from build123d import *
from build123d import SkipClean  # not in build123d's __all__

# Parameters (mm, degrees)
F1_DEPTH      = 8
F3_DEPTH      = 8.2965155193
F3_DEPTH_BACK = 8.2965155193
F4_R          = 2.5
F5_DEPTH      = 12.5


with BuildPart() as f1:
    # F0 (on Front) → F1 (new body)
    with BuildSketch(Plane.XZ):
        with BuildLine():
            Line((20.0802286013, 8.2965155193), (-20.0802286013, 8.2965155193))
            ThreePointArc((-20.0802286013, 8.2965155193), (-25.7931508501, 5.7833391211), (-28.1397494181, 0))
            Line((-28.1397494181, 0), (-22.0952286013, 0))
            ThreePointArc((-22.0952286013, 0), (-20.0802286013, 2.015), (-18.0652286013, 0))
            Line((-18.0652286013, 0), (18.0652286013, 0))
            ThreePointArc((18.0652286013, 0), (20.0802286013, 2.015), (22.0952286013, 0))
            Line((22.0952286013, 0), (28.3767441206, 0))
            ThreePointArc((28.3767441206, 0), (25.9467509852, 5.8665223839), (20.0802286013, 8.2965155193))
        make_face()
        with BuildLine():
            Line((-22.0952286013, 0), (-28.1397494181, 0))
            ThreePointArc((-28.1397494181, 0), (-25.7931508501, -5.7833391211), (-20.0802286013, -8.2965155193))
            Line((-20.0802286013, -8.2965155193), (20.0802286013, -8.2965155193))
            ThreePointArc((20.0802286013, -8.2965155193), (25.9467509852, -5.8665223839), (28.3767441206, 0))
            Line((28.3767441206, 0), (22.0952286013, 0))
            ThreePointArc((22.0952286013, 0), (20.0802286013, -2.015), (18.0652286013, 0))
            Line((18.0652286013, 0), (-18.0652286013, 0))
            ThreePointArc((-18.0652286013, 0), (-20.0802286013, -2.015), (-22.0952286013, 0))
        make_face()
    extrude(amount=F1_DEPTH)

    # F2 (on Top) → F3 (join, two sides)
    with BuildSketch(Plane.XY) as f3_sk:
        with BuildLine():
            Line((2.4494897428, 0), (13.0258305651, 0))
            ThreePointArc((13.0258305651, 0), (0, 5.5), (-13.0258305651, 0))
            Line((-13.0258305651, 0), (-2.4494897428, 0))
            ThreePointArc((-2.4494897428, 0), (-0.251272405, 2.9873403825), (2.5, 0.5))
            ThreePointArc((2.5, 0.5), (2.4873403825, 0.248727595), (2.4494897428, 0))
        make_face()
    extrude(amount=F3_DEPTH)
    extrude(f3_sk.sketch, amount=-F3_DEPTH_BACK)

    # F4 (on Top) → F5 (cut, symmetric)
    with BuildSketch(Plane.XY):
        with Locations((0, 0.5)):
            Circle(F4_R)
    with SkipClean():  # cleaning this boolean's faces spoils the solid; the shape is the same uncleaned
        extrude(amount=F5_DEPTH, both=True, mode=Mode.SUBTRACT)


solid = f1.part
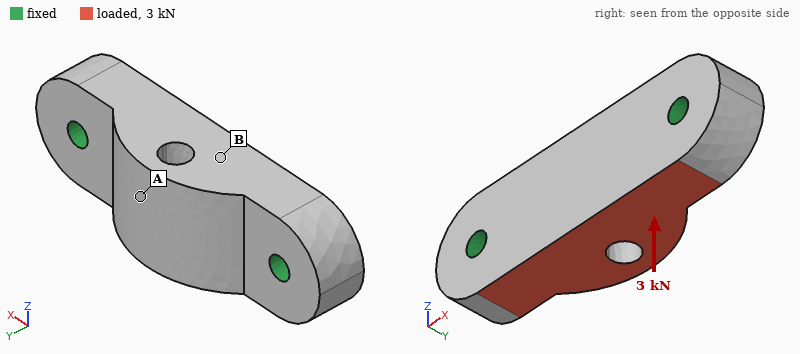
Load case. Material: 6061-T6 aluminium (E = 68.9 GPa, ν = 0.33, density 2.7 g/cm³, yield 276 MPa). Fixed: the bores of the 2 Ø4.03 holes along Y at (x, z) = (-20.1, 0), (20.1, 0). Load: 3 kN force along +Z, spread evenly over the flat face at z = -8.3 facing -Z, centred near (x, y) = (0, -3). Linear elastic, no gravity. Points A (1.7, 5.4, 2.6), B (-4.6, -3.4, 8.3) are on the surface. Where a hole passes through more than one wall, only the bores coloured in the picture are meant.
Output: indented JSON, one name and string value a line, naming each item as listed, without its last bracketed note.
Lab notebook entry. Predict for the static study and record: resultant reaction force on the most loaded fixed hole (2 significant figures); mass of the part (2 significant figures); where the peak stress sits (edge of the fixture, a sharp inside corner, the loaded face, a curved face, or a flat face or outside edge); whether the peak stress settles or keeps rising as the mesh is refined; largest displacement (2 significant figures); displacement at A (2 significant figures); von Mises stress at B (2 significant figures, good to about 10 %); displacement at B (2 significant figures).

{
  "resultant reaction force on the most loaded fixed hole": "1.5 kN",
  "mass of the part": "22 g",
  "where the peak stress sits": "edge of the fixture",
  "whether the peak stress settles or keeps rising as the mesh is refined": "keeps rising",
  "largest displacement": "17 µm",
  "displacement at A": "15 µm",
  "von Mises stress at B": "25 MPa",
  "displacement at B": "10 µm"
}
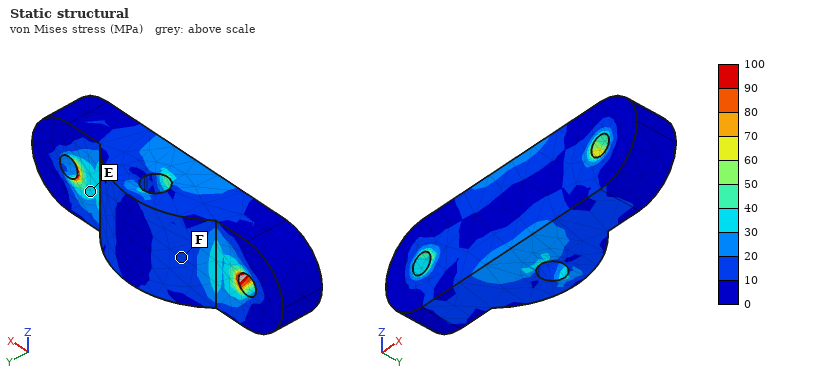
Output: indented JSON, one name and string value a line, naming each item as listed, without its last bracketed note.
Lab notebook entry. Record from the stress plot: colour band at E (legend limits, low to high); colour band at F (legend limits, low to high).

{
  "colour band at E": "30 to 40 MPa",
  "colour band at F": "10 to 20 MPa"
}
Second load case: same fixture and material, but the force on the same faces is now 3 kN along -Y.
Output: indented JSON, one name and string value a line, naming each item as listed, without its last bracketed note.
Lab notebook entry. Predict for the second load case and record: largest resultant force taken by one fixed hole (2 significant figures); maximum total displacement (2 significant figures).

{
  "largest resultant force taken by one fixed hole": "1.5 kN",
  "maximum total displacement": "37 µm"
}
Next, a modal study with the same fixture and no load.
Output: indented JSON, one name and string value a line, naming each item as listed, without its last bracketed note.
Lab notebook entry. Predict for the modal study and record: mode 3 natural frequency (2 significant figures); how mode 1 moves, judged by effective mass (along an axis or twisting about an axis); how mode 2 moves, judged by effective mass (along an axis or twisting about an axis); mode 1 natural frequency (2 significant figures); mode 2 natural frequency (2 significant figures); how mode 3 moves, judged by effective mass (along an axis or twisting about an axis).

{
  "mode 3 natural frequency": "26 kHz",
  "how mode 1 moves, judged by effective mass": "along Z",
  "how mode 2 moves, judged by effective mass": "along Y",
  "mode 1 natural frequency": "19 kHz",
  "mode 2 natural frequency": "21 kHz",
  "how mode 3 moves, judged by effective mass": "along Z"
}
